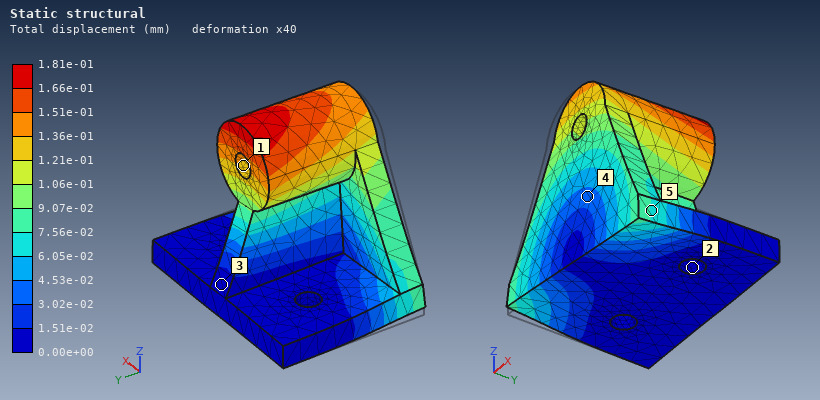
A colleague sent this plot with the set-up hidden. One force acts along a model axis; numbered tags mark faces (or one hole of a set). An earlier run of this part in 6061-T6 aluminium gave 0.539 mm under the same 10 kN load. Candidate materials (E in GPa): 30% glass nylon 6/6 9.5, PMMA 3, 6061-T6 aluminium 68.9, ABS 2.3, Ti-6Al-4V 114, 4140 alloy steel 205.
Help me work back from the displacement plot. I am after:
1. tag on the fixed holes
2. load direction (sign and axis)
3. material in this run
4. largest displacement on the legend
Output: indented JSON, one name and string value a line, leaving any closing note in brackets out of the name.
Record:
{
  "tag on the fixed holes": "2",
  "load direction": "+X",
  "material in this run": "4140 alloy steel",
  "largest displacement on the legend": "1.81e-01 mm"
}
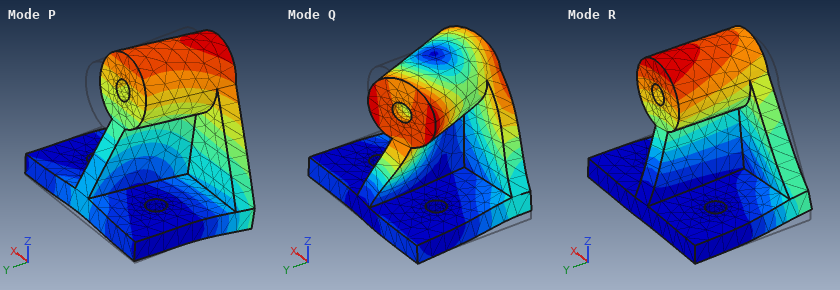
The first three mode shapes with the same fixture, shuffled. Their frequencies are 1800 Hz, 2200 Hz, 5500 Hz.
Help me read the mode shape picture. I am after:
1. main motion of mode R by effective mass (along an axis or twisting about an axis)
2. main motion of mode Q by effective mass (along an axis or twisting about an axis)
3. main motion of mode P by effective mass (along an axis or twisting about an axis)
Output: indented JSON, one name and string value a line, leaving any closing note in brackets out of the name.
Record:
{
  "main motion of mode R by effective mass": "along X",
  "main motion of mode Q by effective mass": "twisting about Z",
  "main motion of mode P by effective mass": "along Y"
}
